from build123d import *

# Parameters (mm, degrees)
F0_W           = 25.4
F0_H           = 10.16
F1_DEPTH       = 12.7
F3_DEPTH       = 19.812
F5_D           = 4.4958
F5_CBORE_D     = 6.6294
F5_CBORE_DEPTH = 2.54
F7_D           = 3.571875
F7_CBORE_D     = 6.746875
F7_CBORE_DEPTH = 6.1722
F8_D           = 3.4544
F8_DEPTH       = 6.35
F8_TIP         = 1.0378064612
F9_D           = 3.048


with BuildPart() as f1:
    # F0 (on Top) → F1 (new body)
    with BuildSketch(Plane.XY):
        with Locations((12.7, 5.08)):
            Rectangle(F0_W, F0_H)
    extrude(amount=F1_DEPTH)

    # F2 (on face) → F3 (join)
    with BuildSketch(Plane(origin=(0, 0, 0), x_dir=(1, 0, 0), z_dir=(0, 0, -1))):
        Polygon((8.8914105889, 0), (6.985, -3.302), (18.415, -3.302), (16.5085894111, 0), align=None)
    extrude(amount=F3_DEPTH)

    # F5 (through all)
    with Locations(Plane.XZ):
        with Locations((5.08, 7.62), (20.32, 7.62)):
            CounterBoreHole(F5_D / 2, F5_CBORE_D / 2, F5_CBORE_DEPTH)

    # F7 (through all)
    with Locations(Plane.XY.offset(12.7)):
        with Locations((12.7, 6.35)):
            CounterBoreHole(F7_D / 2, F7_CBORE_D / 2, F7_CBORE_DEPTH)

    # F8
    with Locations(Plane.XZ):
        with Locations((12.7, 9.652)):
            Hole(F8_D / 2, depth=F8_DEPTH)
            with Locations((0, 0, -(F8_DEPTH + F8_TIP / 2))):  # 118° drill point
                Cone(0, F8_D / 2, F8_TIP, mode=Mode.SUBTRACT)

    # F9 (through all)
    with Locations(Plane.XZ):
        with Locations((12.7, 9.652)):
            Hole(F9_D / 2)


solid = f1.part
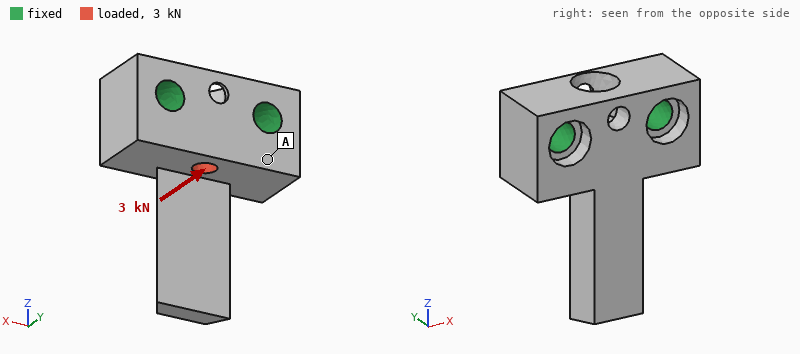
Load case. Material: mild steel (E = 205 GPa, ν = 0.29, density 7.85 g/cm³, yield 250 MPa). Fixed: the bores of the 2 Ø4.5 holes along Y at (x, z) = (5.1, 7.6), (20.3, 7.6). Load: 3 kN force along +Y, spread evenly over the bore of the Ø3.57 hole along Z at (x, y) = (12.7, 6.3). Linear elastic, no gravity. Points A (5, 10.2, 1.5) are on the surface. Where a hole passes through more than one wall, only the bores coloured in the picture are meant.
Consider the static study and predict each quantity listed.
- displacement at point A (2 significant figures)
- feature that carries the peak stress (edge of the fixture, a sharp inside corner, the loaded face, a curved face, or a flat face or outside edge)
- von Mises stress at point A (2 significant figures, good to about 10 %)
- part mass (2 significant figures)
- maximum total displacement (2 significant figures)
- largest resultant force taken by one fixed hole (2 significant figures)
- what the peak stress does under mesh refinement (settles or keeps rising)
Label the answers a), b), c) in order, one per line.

a) 1.3 µm
b) edge of the fixture
c) 15 MPa
d) 25 g
e) 8.7 µm
f) 1.5 kN
g) keeps rising
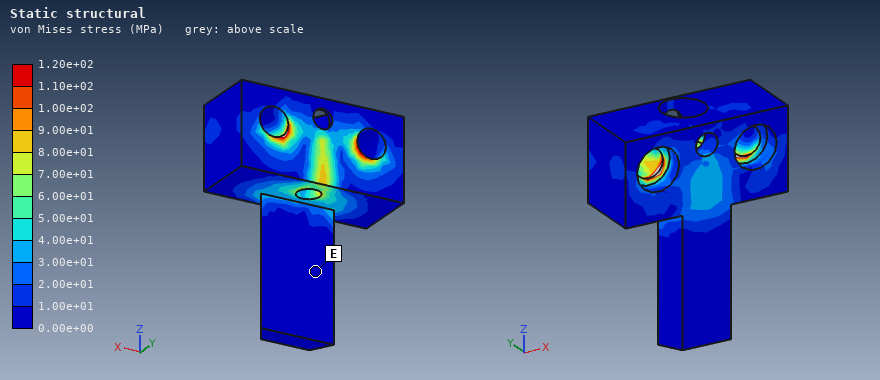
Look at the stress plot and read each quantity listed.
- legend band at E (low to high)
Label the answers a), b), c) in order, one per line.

a) 0.00e+00 to 1.00e+01 MPa
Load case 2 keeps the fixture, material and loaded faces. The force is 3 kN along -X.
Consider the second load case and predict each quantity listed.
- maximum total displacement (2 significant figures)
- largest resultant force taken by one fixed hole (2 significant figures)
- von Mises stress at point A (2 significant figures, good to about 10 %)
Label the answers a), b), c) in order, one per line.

a) 1.6 µm
b) 1.6 kN
c) 12 MPa
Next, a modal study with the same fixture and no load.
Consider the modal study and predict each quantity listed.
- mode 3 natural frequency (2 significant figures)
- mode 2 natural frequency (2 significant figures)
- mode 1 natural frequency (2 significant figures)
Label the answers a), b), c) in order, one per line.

a) 23 kHz
b) 14 kHz
c) 5700 Hz
